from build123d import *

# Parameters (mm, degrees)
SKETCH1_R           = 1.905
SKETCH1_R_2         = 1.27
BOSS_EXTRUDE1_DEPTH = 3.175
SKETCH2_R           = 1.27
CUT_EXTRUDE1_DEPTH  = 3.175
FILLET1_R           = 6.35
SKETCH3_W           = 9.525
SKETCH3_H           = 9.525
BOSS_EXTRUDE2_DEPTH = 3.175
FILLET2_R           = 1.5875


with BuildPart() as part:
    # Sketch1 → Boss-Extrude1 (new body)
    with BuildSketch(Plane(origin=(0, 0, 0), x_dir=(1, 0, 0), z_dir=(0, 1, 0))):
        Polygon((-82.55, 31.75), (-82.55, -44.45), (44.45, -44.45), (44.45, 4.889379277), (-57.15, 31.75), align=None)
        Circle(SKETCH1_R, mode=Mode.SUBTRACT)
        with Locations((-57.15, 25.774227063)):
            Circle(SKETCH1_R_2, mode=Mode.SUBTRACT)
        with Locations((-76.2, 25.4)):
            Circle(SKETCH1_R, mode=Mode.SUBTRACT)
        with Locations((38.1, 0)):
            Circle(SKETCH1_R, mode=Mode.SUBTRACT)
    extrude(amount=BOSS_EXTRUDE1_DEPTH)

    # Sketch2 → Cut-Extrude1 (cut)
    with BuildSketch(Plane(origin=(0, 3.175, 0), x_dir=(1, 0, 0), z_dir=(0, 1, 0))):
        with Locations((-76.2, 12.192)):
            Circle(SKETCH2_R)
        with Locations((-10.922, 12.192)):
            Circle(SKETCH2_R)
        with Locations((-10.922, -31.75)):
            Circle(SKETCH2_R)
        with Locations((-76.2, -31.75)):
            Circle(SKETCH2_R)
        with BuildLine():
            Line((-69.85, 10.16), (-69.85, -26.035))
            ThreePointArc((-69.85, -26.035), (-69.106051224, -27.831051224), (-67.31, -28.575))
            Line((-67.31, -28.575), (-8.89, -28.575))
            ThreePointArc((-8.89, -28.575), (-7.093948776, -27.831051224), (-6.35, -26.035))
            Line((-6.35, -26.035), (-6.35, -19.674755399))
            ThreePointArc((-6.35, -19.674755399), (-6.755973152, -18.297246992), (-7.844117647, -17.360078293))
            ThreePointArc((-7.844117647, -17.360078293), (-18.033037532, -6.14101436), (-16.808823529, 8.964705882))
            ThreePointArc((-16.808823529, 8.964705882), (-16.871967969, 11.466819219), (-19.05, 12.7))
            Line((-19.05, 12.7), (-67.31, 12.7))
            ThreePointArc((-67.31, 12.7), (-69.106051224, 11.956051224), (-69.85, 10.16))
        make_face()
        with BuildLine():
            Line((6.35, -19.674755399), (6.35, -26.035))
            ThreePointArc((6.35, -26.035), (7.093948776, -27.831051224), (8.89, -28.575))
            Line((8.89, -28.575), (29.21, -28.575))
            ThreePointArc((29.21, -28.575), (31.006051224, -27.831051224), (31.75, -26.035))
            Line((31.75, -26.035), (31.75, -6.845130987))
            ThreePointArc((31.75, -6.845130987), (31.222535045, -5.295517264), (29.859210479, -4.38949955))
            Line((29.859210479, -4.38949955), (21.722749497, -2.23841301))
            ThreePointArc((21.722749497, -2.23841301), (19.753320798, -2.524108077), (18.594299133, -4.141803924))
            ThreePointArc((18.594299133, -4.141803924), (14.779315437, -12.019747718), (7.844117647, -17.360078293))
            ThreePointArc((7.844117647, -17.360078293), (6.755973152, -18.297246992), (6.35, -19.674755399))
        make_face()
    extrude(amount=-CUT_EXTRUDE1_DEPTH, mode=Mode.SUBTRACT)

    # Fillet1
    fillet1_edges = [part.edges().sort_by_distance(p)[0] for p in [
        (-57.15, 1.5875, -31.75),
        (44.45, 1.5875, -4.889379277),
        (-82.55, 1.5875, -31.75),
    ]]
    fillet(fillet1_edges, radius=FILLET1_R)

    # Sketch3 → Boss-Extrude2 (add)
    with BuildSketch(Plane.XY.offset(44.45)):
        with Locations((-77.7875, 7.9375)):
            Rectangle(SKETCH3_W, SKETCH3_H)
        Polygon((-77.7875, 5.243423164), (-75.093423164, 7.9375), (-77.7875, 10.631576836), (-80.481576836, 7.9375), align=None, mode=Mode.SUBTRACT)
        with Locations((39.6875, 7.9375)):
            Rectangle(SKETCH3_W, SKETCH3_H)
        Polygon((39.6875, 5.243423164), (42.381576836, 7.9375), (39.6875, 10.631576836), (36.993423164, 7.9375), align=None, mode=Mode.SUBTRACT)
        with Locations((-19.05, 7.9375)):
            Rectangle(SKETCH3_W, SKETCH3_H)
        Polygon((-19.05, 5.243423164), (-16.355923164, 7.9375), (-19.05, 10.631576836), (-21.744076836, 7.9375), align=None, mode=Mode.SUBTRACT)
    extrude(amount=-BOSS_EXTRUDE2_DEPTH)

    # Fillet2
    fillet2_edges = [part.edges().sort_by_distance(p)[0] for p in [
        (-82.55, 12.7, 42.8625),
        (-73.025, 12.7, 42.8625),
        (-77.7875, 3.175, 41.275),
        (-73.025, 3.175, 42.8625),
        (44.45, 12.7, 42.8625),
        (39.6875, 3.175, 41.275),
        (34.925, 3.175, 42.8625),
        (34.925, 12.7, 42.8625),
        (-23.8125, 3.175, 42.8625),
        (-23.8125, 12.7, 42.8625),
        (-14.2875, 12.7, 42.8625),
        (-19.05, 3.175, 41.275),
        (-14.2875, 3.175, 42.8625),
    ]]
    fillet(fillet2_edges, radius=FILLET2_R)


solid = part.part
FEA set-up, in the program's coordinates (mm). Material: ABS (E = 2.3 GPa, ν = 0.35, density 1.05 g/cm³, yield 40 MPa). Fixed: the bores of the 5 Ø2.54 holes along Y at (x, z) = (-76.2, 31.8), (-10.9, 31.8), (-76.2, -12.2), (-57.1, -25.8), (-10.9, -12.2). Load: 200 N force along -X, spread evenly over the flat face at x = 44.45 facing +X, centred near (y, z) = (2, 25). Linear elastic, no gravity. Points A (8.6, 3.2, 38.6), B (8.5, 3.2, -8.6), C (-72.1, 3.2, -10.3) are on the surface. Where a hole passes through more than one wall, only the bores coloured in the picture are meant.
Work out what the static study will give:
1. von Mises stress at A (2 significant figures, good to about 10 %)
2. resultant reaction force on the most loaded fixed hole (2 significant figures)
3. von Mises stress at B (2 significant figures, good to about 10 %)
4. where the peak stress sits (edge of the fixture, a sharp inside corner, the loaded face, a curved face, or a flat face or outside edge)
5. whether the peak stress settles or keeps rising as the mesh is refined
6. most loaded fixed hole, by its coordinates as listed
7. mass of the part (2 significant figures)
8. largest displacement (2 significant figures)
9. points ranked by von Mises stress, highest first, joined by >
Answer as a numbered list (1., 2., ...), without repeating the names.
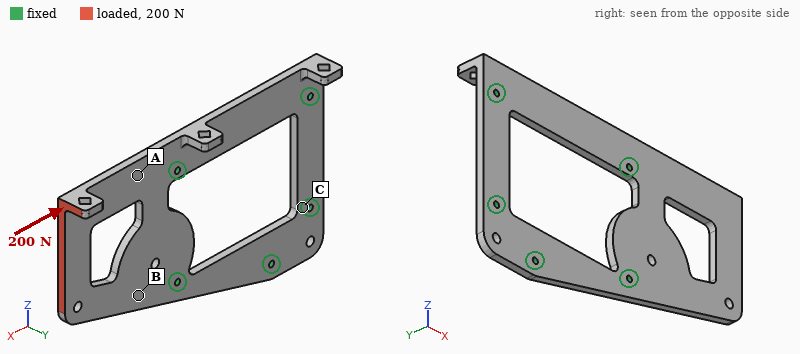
1. 6.2 MPa
2. 140 N
3. 2.7 MPa
4. edge of the fixture
5. keeps rising
6. (-10.9, 31.8)
7. 19 g
8. 1.7 mm
9. A > B > C
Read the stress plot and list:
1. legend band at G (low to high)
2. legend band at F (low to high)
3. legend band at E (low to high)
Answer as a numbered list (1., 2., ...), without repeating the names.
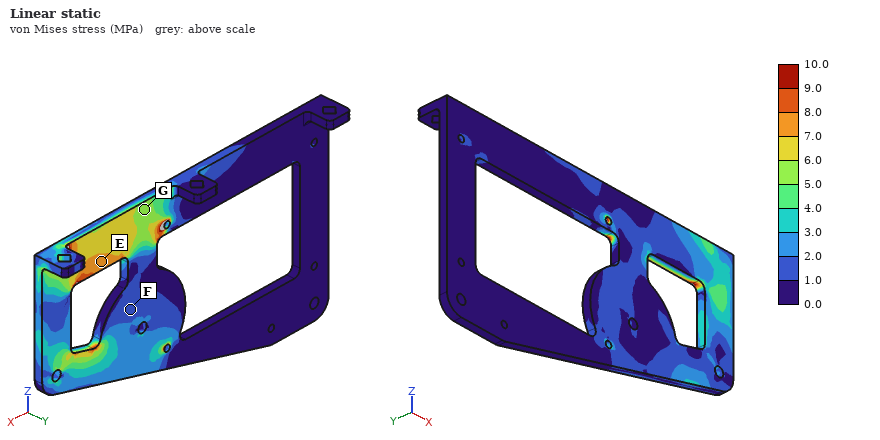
1. 5.0 to 6.0 MPa
2. 1.0 to 2.0 MPa
3. 7.0 to 8.0 MPa
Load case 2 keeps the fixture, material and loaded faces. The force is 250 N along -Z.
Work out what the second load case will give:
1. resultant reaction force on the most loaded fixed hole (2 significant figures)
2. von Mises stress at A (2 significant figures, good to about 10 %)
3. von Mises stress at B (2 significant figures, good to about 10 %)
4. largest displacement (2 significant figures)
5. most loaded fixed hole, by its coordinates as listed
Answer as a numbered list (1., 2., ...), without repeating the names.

1. 310 N
2. 7.0 MPa
3. 5.8 MPa
4. 1.5 mm
5. (-10.9, -12.2)
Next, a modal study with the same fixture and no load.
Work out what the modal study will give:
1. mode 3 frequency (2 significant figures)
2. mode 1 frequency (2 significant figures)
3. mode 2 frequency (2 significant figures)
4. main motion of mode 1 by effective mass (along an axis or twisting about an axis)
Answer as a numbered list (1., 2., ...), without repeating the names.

1. 1000 Hz
2. 210 Hz
3. 520 Hz
4. along Y
